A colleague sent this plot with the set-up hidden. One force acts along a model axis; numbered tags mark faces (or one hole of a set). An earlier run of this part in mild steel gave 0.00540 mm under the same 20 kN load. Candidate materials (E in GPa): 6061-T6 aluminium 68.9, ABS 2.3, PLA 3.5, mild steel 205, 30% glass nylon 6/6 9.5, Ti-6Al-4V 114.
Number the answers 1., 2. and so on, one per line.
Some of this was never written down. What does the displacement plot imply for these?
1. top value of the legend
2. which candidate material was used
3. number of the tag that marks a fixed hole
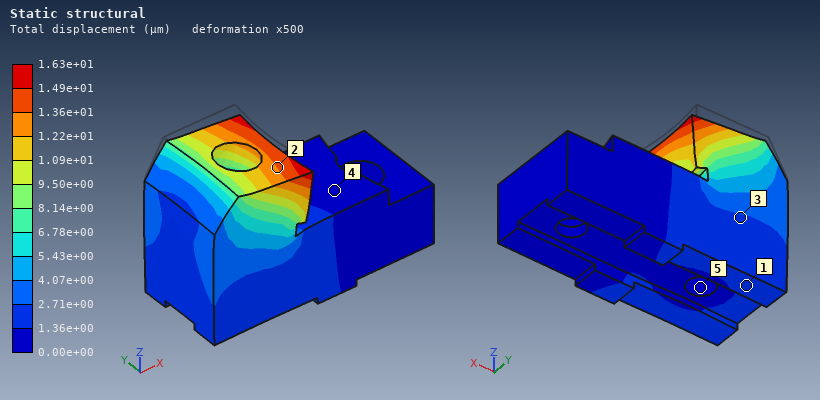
1. 1.63e+01 µm
2. 6061-T6 aluminium
3. 5
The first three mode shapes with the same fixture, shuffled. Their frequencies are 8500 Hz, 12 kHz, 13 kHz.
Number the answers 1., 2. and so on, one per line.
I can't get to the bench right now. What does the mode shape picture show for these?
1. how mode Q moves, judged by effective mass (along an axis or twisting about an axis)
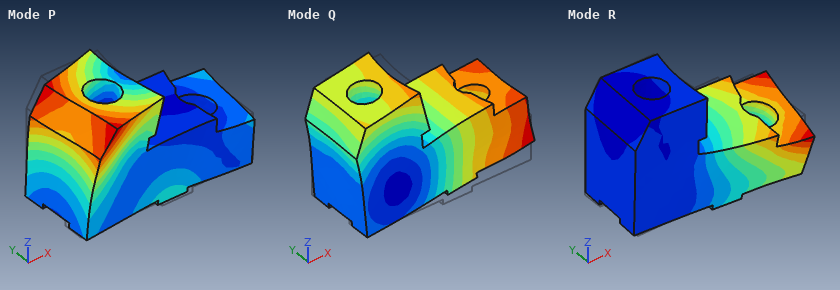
1. along Z
